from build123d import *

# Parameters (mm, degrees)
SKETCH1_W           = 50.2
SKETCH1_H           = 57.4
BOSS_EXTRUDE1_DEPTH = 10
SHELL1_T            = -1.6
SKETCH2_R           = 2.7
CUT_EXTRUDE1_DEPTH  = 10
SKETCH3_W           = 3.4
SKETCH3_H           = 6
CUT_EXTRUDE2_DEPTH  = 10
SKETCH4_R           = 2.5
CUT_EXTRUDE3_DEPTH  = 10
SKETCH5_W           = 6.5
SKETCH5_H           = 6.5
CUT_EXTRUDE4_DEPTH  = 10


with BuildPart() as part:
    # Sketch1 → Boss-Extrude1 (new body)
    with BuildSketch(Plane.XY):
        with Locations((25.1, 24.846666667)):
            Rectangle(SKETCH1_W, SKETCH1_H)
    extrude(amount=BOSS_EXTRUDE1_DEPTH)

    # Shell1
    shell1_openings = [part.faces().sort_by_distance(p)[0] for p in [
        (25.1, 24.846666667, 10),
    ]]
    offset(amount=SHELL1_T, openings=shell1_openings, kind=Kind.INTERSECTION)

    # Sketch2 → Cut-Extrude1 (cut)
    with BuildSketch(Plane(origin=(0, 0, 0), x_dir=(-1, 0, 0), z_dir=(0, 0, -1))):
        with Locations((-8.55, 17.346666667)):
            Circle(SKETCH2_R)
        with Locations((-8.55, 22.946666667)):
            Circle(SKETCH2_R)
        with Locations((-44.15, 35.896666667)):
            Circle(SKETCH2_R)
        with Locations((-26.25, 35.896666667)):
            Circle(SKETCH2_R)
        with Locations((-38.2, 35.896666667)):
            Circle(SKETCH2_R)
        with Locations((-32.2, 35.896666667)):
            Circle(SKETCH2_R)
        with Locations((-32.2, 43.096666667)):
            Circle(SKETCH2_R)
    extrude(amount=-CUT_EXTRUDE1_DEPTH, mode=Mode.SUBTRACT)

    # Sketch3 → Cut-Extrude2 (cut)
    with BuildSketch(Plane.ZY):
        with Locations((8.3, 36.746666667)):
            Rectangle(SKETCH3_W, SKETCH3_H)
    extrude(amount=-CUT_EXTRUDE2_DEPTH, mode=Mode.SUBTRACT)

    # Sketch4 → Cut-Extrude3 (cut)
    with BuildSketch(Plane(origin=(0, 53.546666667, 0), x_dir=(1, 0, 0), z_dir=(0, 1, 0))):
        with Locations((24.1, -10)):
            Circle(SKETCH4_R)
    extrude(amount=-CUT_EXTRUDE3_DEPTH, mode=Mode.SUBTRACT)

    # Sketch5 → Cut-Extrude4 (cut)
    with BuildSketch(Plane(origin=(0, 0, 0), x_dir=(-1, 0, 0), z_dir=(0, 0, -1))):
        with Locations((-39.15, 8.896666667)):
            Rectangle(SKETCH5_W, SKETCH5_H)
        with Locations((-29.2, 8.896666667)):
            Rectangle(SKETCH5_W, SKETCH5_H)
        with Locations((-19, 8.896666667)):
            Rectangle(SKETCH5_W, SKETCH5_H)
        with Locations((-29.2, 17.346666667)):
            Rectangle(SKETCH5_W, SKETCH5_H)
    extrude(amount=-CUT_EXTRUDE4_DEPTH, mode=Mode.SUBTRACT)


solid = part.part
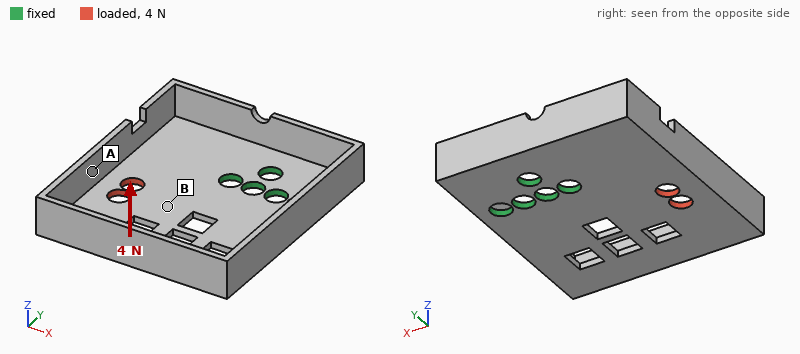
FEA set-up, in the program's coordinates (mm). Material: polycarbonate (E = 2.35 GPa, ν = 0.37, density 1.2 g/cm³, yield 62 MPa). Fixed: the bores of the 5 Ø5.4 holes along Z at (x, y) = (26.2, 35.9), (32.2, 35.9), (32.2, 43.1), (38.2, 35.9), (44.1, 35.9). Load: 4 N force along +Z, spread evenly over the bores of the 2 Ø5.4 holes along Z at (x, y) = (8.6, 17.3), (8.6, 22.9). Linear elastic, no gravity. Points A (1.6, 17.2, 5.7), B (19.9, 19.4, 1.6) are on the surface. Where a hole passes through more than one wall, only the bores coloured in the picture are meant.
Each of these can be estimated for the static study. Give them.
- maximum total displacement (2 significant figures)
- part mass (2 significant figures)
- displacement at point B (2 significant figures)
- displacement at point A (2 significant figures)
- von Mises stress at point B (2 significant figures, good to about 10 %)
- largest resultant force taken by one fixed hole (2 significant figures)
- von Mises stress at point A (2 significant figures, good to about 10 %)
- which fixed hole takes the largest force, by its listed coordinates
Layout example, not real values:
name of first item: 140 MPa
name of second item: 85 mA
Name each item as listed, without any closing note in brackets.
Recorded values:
maximum total displacement: 0.75 mm
part mass: 8.2 g
displacement at point B: 0.19 mm
displacement at point A: 0.46 mm
von Mises stress at point B: 0.91 MPa
largest resultant force taken by one fixed hole: 6.7 N
von Mises stress at point A: 0.40 MPa
which fixed hole takes the largest force, by its listed coordinates: (26.2, 35.9)
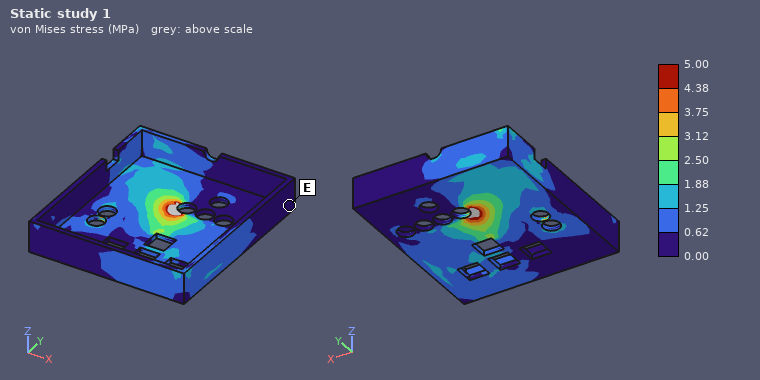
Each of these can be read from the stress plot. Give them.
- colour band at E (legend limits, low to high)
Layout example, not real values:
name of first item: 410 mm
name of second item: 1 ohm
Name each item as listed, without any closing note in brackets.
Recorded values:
colour band at E: 0.00 to 0.62 MPa
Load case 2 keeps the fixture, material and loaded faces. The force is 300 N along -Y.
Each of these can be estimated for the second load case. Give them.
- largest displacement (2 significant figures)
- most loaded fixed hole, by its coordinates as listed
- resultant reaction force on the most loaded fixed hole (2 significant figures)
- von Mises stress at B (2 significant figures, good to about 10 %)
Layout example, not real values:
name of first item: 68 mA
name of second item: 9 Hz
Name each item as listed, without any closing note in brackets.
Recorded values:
largest displacement: 0.50 mm
most loaded fixed hole, by its coordinates as listed: (26.2, 35.9)
resultant reaction force on the most loaded fixed hole: 400 N
von Mises stress at B: 5.7 MPa
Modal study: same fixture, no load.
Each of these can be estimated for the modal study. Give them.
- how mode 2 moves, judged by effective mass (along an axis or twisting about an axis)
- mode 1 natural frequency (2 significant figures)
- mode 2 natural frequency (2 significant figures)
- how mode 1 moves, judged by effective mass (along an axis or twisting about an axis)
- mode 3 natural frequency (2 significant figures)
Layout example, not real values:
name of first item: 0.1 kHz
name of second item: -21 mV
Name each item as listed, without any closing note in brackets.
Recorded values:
how mode 2 moves, judged by effective mass: along Z
mode 1 natural frequency: 230 Hz
mode 2 natural frequency: 550 Hz
how mode 1 moves, judged by effective mass: along Z
mode 3 natural frequency: 660 Hz
